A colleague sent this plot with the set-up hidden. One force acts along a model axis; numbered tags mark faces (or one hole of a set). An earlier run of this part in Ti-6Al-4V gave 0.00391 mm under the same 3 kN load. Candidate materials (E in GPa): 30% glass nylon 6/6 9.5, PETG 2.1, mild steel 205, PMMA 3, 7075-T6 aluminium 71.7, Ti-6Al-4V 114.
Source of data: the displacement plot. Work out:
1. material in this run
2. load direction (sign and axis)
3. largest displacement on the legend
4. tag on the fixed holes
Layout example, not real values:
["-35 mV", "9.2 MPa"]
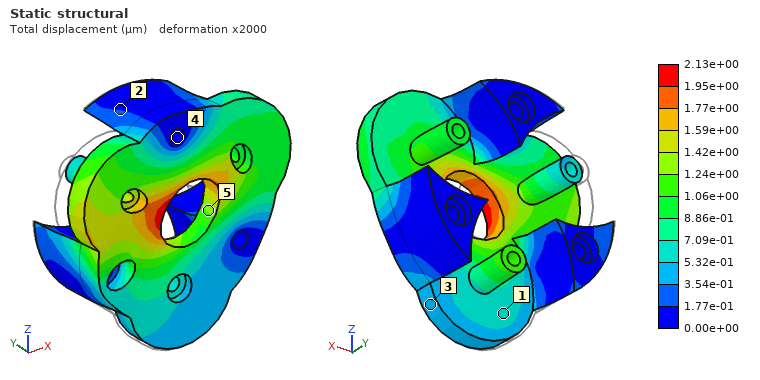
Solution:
["mild steel", "+X", "2.13e+00 µm", "4"]
